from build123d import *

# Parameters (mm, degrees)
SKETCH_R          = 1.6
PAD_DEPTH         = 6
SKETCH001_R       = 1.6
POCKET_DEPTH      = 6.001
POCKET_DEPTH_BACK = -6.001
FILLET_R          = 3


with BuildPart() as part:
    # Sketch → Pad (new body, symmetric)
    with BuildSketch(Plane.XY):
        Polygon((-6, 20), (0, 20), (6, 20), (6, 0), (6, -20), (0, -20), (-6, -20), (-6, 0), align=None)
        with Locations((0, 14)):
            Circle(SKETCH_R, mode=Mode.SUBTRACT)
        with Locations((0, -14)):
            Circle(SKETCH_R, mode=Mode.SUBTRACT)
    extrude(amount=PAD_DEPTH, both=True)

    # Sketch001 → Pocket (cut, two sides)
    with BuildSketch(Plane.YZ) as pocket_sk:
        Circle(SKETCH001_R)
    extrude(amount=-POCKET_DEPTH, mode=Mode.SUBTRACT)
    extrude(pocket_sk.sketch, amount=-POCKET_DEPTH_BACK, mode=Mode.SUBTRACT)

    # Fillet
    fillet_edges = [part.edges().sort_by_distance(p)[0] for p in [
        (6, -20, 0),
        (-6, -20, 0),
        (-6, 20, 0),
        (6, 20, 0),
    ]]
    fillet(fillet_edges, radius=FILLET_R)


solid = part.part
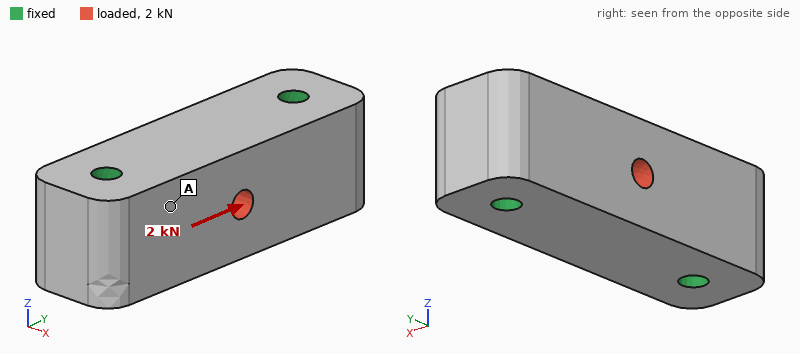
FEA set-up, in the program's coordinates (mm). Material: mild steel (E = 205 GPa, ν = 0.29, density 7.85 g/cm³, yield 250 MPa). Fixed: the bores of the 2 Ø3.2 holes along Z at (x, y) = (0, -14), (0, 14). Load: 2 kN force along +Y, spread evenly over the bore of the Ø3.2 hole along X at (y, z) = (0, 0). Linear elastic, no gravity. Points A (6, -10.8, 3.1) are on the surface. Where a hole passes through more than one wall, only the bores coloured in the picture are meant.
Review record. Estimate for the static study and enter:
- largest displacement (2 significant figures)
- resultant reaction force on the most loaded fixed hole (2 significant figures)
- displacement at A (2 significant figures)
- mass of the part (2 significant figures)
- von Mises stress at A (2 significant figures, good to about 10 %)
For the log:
0.65 µm
1.0 kN
0.22 µm
42 g
3.8 MPa
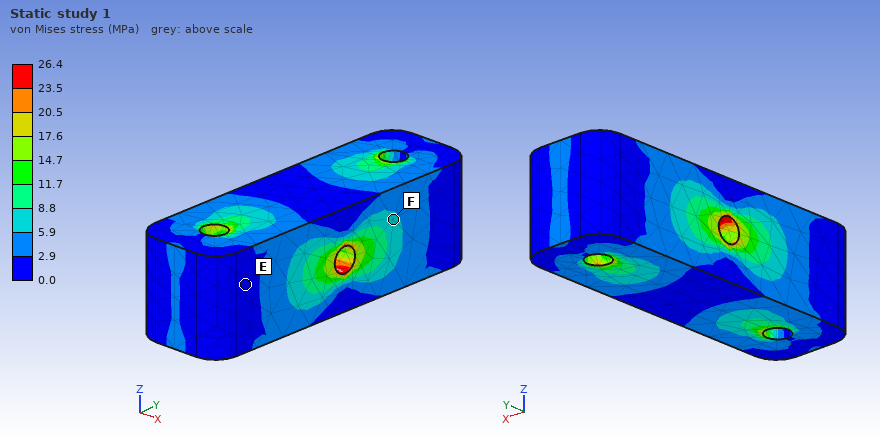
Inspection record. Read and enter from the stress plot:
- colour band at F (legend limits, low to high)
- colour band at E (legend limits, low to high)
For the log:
5.9 to 8.8 MPa
0.0 to 2.9 MPa
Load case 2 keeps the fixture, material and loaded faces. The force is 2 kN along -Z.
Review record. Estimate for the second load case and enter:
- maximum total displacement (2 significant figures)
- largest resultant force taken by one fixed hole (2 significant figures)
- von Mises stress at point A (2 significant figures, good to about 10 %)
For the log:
2.2 µm
1.0 kN
8.7 MPa
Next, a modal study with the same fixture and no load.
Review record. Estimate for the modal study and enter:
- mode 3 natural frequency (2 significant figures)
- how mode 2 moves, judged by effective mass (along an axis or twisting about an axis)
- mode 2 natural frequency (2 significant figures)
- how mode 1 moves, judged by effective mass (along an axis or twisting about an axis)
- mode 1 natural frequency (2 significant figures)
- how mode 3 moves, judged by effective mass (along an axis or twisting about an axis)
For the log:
52 kHz
along Z
44 kHz
along X
36 kHz
twisting about Y
